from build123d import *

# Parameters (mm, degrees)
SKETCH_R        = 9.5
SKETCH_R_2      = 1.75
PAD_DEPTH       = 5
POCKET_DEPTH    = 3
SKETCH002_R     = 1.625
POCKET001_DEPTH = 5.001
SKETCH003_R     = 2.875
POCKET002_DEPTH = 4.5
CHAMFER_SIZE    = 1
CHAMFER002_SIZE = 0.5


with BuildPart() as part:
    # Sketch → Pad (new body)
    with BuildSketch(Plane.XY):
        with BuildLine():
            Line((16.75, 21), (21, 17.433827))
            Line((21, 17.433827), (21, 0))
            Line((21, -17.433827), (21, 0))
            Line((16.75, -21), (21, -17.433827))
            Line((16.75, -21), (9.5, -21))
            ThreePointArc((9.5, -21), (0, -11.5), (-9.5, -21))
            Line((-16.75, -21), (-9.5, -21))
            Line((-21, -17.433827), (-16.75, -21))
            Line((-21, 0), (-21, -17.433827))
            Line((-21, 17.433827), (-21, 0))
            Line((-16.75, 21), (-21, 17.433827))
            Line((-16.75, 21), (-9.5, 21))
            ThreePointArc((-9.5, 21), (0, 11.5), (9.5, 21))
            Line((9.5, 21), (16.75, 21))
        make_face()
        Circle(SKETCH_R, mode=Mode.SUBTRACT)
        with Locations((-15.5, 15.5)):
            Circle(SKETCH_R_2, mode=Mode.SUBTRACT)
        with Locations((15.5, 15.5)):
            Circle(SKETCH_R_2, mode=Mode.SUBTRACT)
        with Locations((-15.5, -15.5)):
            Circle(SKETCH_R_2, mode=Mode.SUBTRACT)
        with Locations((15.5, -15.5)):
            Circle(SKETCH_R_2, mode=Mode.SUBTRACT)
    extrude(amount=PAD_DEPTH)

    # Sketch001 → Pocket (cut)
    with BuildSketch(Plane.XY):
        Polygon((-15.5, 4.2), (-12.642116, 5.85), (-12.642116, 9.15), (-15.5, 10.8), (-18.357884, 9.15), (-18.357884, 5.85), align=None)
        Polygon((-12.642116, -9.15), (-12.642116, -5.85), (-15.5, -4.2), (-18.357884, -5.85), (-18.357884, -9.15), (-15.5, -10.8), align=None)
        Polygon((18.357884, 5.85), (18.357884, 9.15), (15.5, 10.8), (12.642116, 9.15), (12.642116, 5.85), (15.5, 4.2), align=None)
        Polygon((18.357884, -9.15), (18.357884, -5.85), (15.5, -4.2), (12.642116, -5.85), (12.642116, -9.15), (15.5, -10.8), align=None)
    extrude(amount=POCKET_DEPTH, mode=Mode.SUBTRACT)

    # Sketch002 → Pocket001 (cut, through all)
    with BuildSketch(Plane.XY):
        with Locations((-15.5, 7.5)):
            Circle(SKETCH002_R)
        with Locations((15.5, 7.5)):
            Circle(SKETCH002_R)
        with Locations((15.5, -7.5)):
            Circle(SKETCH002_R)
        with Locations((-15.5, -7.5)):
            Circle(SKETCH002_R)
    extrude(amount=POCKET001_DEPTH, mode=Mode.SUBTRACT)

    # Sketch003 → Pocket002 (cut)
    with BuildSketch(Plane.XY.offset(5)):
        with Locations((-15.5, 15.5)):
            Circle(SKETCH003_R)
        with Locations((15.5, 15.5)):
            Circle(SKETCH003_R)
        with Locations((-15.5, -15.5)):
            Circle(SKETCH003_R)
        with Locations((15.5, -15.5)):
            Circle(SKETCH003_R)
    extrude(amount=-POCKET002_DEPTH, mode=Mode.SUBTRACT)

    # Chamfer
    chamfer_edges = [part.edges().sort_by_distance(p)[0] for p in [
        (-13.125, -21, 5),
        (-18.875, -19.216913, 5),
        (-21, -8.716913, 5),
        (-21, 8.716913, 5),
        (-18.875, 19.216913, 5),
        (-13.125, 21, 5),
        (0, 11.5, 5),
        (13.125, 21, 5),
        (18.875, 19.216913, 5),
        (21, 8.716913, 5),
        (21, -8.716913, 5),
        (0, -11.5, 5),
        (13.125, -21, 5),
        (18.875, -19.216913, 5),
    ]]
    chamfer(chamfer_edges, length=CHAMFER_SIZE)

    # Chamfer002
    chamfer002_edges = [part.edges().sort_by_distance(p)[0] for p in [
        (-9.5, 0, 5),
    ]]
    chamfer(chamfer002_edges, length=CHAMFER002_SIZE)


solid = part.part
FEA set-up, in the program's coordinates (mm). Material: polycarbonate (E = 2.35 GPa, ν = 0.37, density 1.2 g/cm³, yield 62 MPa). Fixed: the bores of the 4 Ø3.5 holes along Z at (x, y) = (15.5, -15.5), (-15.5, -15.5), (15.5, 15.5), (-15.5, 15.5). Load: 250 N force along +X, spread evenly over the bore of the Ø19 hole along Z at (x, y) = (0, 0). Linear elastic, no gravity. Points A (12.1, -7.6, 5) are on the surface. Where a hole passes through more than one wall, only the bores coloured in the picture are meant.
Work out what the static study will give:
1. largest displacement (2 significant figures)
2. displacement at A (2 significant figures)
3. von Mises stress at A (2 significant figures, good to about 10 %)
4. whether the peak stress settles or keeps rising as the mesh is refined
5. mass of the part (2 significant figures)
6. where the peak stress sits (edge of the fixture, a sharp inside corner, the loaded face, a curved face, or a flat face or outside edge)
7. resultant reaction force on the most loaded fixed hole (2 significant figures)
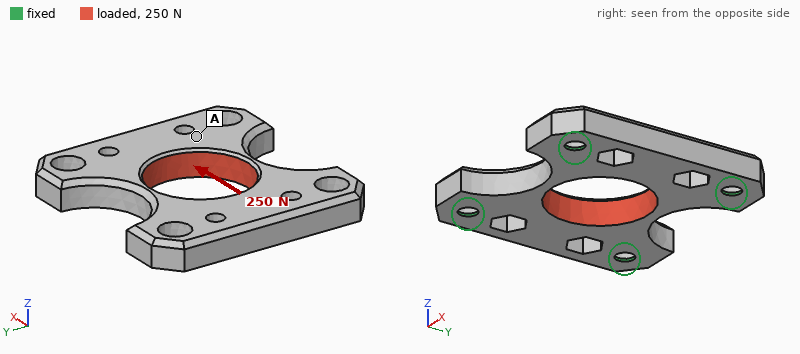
58 µm
45 µm
2.1 MPa
keeps rising
5.8 g
edge of the fixture
65 N
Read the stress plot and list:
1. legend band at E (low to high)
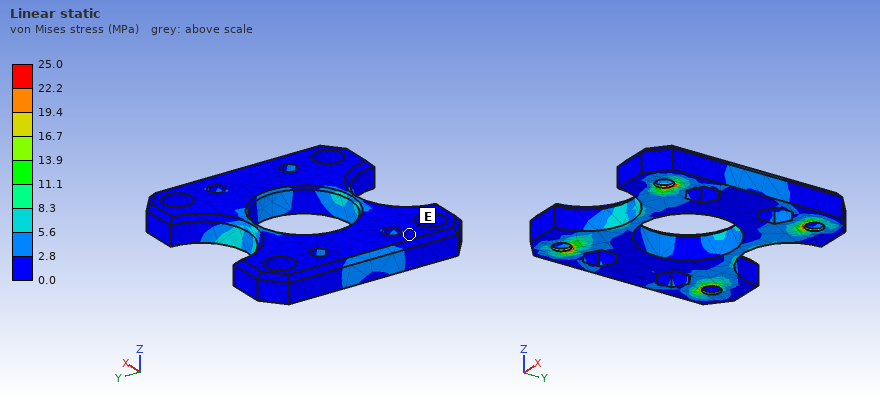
0.0 to 2.8 MPa
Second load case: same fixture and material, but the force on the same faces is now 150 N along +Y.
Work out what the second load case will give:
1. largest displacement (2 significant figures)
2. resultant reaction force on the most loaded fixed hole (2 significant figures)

39 µm
41 N
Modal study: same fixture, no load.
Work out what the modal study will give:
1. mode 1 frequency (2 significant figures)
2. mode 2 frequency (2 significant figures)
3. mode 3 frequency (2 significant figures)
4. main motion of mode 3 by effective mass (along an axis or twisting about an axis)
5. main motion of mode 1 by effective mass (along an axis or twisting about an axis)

3000 Hz
3700 Hz
4000 Hz
along Z
along Z
